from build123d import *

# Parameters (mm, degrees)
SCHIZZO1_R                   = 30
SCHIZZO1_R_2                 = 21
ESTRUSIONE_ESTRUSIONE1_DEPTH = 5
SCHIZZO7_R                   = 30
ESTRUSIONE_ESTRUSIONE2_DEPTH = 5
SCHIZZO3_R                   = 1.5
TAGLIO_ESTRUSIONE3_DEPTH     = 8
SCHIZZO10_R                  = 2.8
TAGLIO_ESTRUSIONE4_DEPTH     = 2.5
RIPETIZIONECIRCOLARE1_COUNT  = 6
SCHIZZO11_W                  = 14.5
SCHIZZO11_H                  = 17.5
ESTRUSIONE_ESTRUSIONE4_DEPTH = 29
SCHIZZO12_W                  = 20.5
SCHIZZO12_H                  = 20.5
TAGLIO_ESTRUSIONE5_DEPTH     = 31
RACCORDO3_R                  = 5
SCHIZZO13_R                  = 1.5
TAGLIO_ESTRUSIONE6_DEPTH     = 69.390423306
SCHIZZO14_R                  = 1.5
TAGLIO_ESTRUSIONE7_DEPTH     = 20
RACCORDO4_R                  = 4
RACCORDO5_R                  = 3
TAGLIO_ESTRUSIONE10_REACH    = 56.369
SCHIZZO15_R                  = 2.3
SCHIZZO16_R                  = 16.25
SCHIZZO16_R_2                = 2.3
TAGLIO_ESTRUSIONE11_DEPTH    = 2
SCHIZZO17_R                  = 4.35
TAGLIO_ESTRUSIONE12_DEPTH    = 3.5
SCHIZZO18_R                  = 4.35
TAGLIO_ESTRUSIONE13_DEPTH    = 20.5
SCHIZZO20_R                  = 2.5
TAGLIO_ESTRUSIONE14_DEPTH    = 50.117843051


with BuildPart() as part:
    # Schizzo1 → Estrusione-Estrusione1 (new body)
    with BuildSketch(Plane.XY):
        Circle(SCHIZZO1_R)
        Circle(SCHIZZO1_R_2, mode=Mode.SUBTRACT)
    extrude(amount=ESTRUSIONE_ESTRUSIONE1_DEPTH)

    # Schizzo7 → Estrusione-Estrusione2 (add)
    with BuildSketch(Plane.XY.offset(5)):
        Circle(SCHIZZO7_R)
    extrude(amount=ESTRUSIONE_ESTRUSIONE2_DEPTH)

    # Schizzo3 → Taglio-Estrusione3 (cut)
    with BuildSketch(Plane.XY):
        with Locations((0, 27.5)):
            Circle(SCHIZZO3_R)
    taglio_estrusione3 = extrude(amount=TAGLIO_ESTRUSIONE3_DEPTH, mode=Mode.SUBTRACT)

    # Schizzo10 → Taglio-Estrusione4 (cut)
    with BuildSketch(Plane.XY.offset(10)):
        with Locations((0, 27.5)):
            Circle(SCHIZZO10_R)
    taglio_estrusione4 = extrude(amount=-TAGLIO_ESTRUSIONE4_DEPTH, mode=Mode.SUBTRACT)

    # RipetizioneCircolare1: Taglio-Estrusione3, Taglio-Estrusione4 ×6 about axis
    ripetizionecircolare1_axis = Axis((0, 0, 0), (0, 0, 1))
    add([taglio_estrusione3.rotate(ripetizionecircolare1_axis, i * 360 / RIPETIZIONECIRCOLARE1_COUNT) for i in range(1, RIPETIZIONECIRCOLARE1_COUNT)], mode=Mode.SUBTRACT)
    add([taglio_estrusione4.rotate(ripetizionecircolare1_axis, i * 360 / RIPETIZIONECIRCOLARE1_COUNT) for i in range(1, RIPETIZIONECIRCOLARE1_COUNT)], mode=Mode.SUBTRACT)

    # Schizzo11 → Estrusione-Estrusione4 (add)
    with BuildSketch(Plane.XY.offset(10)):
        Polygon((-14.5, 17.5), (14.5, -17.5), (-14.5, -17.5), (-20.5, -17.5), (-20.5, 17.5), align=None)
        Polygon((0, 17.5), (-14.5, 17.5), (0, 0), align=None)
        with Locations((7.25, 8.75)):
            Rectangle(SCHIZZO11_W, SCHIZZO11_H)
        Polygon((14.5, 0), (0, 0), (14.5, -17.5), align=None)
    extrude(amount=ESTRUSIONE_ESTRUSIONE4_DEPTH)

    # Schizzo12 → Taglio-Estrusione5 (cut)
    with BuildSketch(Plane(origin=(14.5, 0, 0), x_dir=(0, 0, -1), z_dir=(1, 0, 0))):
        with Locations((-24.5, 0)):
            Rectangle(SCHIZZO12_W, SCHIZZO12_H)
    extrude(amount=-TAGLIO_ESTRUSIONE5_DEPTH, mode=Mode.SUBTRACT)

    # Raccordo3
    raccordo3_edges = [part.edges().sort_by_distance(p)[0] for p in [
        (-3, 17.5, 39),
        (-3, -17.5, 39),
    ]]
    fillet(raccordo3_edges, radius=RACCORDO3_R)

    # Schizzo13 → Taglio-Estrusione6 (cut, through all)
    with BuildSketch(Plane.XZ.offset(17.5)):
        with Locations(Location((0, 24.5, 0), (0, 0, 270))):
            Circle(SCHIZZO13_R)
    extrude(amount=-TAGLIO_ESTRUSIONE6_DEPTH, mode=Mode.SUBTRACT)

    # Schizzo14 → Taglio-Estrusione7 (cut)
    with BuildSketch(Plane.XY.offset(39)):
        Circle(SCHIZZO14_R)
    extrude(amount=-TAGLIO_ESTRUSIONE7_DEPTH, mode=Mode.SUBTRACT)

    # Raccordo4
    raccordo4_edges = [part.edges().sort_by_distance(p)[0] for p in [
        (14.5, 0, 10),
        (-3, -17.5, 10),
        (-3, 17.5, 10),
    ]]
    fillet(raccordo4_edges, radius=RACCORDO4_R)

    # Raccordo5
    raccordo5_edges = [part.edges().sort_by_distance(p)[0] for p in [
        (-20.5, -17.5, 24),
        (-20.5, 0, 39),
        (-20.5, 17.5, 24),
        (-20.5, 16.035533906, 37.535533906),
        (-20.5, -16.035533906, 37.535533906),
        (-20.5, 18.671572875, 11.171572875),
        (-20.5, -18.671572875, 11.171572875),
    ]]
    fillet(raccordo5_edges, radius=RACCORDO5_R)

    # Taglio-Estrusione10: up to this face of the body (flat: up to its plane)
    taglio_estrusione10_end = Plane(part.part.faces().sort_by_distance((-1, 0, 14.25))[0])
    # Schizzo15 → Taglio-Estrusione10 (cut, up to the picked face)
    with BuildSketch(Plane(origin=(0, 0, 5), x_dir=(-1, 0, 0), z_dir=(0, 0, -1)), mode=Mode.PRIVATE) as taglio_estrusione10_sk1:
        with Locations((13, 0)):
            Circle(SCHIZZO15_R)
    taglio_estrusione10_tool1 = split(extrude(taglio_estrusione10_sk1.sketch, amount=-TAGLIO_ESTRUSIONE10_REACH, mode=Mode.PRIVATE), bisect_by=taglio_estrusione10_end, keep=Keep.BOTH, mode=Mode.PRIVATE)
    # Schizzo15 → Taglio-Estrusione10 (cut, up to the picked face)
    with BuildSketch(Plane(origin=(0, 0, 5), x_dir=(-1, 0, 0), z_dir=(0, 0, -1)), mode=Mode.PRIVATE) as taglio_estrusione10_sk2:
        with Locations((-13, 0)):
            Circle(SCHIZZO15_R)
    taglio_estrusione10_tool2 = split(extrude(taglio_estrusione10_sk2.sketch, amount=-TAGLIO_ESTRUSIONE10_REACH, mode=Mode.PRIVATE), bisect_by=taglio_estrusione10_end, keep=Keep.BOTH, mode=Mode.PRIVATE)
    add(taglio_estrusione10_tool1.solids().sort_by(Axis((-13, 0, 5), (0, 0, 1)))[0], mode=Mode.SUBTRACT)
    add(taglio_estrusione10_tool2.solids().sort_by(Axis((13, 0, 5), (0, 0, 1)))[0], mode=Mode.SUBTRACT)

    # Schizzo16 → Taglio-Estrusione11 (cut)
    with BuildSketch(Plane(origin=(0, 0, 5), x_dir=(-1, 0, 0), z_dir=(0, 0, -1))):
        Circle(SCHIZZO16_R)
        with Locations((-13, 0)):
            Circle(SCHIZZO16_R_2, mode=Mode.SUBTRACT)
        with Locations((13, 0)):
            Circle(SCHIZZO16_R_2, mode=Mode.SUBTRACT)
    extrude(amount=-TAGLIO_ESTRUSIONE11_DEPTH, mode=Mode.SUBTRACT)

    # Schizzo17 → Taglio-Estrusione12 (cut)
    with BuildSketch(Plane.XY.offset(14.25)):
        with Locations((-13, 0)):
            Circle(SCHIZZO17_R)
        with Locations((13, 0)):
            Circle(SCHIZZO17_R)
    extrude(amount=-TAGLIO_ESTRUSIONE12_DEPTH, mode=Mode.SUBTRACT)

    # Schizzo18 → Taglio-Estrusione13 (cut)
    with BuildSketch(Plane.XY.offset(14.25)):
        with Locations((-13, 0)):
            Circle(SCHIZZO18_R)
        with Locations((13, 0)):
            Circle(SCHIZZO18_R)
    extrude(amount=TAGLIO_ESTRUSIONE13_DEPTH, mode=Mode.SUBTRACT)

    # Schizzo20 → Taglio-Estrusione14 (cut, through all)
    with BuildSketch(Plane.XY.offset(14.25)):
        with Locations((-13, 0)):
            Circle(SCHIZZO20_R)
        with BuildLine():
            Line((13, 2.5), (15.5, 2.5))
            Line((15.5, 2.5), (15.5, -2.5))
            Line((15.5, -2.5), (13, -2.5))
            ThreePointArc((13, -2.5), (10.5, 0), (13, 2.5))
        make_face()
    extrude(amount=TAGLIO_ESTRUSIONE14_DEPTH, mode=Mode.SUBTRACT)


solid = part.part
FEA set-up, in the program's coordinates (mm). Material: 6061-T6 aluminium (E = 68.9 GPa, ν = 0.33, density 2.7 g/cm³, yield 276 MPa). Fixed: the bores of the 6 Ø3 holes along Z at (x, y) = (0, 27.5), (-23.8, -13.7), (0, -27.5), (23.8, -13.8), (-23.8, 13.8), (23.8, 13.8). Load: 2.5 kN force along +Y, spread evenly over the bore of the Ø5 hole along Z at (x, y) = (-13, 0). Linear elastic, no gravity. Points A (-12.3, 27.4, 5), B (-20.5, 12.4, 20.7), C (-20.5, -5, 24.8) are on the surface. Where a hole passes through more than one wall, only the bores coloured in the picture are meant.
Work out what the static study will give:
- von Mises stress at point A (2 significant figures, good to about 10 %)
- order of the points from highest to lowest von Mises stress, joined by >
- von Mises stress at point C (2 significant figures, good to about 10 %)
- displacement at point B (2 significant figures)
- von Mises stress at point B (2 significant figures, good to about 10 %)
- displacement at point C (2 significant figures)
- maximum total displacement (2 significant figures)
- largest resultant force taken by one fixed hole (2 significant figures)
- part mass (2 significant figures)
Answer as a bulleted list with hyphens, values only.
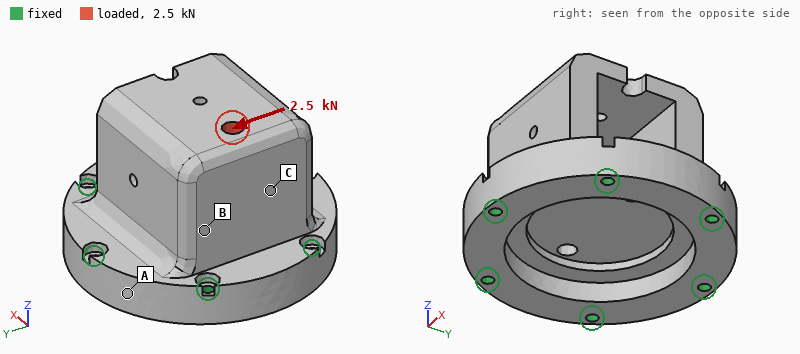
- 7.0 MPa
- C > B > A
- 24 MPa
- 11 µm
- 16 MPa
- 13 µm
- 32 µm
- 1.2 kN
- 110 g
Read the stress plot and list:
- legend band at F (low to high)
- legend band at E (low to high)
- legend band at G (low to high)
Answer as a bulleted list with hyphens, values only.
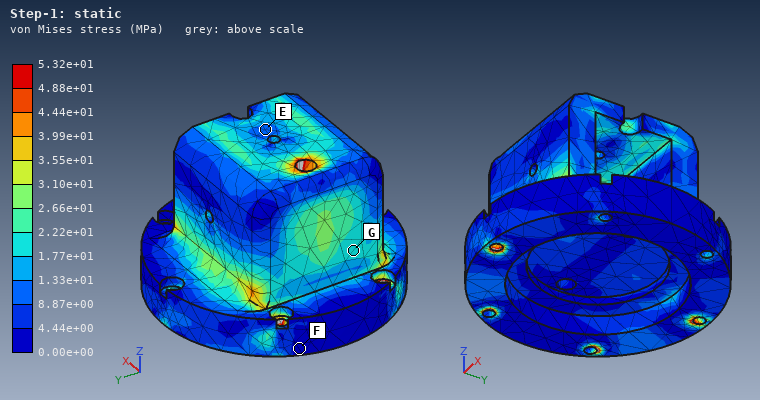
- 0.00e+00 to 4.44e+00 MPa
- 8.87e+00 to 1.33e+01 MPa
- 1.77e+01 to 2.22e+01 MPa
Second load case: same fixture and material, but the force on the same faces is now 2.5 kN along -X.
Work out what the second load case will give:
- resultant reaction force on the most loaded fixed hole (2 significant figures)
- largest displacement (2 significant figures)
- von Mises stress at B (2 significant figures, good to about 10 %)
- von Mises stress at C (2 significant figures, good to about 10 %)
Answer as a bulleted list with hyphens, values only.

- 1.2 kN
- 27 µm
- 11 MPa
- 8.3 MPa
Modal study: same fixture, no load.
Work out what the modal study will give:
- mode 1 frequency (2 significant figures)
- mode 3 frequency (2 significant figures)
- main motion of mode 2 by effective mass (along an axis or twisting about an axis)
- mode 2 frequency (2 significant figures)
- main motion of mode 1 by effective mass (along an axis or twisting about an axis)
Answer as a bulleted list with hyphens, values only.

- 8700 Hz
- 17 kHz
- along X
- 12 kHz
- along Y
